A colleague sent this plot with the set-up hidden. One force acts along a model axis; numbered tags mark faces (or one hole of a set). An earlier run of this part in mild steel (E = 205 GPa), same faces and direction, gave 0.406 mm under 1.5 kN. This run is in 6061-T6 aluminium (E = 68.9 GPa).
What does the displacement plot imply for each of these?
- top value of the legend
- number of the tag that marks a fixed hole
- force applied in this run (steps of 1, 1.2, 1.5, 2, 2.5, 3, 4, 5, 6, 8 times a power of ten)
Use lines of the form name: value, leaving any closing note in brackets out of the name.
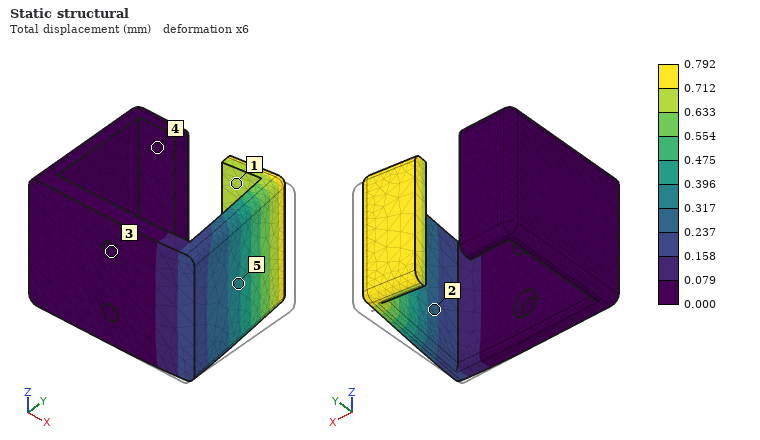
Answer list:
top value of the legend: 0.792 mm
number of the tag that marks a fixed hole: 3
force applied in this run: 1 kN
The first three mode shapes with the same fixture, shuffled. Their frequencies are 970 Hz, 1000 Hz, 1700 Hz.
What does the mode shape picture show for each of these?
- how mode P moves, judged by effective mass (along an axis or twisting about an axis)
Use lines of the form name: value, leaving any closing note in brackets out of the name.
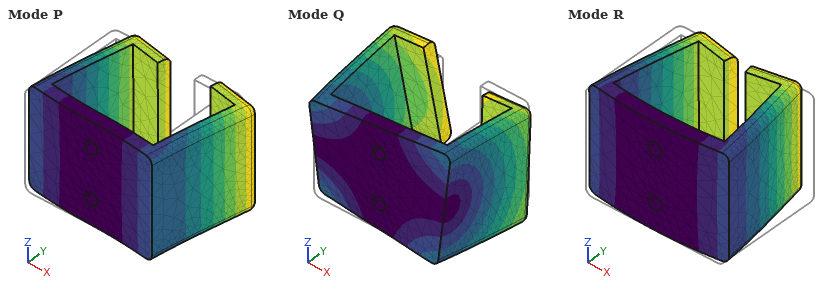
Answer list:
how mode P moves, judged by effective mass: along X
